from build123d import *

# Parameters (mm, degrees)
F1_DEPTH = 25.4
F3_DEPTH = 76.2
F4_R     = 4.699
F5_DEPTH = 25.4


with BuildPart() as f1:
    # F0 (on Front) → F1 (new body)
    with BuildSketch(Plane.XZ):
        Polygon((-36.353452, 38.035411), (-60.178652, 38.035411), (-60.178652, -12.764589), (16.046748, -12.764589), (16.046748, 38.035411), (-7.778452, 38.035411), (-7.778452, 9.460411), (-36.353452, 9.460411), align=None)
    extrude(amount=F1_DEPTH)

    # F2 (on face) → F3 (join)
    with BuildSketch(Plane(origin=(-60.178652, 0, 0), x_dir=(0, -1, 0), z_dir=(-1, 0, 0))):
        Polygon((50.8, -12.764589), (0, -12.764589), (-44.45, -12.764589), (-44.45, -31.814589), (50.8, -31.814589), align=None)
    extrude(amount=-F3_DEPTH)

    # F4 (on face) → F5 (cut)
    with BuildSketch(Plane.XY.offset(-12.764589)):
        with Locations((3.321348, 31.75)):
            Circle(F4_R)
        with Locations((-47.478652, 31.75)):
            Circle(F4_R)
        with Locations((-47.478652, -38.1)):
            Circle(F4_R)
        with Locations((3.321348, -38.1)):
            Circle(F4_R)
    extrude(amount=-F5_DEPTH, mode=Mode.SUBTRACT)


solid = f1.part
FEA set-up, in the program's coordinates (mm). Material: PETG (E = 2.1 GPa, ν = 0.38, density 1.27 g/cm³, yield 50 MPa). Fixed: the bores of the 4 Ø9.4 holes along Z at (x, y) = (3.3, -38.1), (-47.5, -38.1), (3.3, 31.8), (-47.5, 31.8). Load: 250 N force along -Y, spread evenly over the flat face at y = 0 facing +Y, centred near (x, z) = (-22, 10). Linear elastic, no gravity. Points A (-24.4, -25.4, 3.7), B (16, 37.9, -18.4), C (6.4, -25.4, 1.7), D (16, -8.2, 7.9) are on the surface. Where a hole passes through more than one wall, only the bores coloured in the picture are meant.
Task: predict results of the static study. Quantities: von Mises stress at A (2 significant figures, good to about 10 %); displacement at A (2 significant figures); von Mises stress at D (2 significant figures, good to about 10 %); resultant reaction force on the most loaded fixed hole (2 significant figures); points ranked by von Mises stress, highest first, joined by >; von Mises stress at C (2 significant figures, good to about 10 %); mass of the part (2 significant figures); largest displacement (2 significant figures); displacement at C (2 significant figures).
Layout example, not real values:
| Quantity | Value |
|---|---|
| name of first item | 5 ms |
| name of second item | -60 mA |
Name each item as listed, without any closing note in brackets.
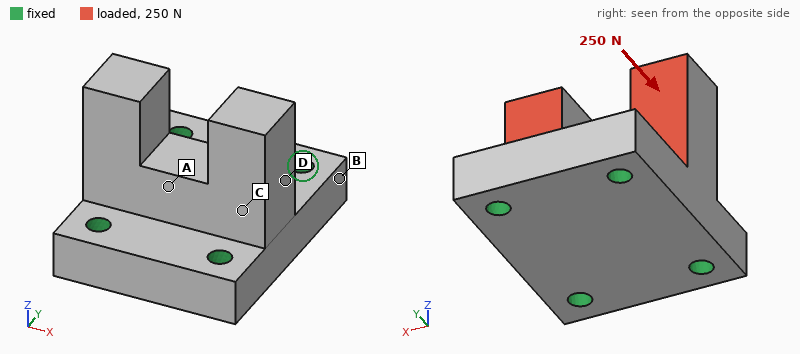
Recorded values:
| Quantity | Value |
|---|---|
| von Mises stress at A | 0.14 MPa |
| displacement at A | 14 µm |
| von Mises stress at D | 0.26 MPa |
| resultant reaction force on the most loaded fixed hole | 100 N |
| points ranked by von Mises stress, highest first, joined by > | C > D > A > B |
| von Mises stress at C | 0.40 MPa |
| mass of the part | 270 g |
| largest displacement | 50 µm |
| displacement at C | 15 µm |
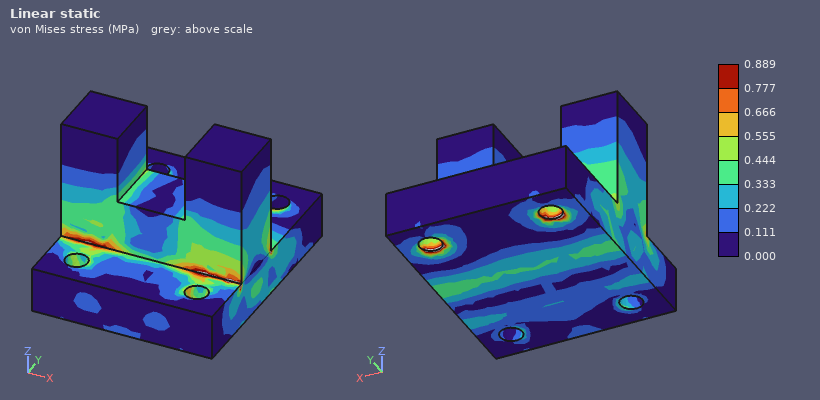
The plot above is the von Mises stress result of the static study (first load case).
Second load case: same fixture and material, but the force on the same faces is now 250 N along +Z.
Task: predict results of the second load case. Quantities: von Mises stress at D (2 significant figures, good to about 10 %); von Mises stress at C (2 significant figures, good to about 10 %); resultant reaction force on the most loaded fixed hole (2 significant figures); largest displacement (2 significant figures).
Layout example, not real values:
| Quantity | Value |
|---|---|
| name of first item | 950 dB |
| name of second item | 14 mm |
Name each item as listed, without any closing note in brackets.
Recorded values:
| Quantity | Value |
|---|---|
| von Mises stress at D | 0.19 MPa |
| von Mises stress at C | 0.19 MPa |
| resultant reaction force on the most loaded fixed hole | 71 N |
| largest displacement | 35 µm |
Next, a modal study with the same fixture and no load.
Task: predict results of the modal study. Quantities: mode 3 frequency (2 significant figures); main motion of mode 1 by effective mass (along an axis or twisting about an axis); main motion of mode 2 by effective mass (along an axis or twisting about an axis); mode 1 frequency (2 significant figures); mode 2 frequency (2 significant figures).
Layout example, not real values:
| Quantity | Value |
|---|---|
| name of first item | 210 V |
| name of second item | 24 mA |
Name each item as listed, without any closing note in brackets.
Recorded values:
| Quantity | Value |
|---|---|
| mode 3 frequency | 1700 Hz |
| main motion of mode 1 by effective mass | along Y |
| main motion of mode 2 by effective mass | along X |
| mode 1 frequency | 1400 Hz |
| mode 2 frequency | 1500 Hz |
